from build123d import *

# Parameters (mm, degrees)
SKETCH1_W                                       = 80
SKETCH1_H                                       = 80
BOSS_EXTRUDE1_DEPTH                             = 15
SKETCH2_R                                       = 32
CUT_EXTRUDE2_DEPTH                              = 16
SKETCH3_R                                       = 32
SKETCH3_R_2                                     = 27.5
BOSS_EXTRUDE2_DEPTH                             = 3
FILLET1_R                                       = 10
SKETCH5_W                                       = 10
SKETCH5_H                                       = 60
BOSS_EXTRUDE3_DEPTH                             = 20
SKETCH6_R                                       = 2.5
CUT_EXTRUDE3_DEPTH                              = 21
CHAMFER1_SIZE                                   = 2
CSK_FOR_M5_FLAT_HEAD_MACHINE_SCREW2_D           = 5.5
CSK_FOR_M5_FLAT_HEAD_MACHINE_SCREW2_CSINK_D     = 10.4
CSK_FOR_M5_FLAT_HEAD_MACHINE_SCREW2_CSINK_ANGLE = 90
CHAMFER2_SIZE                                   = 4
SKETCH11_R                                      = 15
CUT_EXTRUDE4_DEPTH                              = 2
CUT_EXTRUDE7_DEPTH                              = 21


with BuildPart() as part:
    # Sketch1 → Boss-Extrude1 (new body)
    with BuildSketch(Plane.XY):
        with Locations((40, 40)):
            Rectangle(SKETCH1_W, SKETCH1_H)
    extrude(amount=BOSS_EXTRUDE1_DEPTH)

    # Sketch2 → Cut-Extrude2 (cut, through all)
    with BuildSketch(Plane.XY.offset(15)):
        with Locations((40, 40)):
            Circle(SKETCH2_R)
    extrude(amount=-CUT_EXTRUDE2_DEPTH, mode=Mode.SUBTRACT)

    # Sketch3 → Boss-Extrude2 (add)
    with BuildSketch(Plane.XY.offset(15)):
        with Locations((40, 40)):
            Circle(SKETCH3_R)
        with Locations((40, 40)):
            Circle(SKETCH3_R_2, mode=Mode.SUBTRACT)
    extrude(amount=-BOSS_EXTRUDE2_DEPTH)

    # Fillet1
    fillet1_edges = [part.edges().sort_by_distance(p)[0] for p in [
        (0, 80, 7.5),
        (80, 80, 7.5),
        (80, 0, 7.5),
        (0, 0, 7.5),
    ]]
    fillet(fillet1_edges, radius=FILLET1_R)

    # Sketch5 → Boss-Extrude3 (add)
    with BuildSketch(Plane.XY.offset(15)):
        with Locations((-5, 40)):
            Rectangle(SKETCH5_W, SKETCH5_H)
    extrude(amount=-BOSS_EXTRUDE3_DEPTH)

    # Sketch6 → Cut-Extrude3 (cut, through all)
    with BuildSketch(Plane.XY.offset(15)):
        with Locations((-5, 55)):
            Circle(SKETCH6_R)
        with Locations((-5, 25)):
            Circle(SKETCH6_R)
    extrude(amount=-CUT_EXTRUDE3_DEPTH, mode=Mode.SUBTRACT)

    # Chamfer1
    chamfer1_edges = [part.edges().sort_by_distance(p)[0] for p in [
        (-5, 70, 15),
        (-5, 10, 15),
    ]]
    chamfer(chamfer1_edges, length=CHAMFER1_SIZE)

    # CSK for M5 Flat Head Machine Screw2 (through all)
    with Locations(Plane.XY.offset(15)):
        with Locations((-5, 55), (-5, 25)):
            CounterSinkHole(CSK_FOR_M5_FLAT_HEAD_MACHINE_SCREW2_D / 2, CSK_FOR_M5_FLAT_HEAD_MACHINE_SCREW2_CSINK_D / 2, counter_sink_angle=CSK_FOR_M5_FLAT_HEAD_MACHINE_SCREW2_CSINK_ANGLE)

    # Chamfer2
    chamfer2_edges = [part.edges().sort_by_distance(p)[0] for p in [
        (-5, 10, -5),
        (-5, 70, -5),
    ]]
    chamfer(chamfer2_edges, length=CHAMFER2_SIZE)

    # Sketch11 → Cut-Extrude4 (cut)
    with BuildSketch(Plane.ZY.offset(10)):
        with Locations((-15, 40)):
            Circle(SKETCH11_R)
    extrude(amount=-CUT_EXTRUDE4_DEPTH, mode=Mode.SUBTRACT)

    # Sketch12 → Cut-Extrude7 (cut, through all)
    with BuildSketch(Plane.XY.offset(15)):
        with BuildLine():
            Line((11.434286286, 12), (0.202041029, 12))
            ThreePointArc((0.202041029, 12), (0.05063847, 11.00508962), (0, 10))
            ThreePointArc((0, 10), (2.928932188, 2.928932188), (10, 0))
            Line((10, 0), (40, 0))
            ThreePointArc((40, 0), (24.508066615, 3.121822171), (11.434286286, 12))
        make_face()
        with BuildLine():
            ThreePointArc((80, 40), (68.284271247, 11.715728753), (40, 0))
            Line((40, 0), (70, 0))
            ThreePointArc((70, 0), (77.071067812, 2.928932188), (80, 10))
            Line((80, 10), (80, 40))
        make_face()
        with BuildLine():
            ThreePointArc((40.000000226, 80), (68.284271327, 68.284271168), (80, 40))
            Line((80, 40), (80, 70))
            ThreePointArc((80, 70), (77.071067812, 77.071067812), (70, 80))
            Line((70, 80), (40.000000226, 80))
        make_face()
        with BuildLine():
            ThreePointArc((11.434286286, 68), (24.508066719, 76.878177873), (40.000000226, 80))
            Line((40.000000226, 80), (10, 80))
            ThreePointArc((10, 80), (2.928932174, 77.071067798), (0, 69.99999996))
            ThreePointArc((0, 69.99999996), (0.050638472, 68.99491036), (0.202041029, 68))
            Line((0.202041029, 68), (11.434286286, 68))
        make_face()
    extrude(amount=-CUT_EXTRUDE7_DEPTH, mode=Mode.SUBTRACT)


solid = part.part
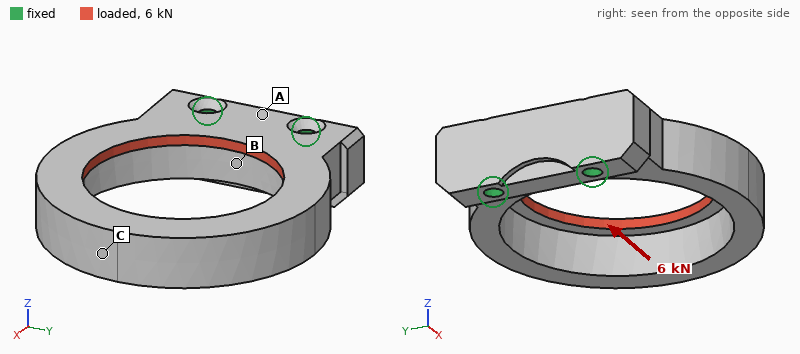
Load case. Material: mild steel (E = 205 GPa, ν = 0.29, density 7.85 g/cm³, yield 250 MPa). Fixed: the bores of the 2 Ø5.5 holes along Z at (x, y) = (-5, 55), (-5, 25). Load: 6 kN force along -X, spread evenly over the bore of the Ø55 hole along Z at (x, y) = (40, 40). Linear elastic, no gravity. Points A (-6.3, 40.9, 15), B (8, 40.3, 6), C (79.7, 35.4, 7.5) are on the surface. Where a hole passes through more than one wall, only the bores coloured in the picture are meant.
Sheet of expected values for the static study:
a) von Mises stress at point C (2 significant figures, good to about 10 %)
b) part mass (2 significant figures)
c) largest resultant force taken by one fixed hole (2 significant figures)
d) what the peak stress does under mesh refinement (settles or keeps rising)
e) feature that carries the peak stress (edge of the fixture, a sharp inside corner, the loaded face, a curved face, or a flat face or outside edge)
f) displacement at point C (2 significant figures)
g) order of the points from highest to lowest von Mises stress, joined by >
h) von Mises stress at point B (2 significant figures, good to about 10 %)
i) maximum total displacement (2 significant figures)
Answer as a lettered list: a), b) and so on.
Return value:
a) 34 MPa
b) 340 g
c) 3.3 kN
d) keeps rising
e) edge of the fixture
f) 79 µm
g) C > B > A
h) 19 MPa
i) 86 µm
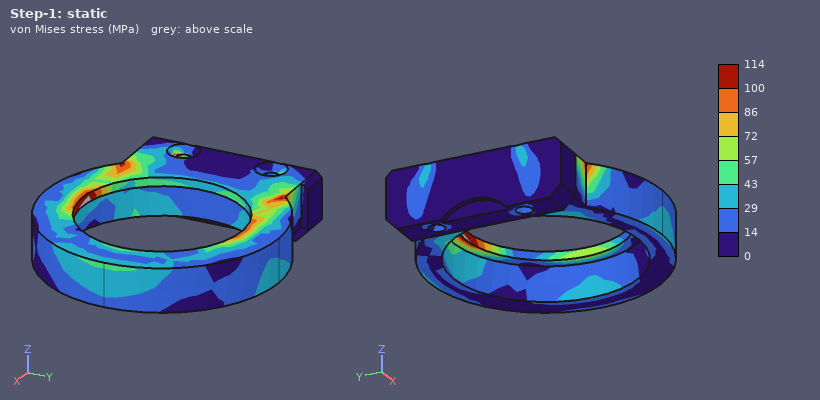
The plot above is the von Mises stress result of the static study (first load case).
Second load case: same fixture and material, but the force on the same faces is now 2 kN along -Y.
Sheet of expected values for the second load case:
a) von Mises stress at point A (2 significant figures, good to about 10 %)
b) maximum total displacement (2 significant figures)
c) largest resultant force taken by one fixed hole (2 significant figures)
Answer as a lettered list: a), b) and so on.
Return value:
a) 8.4 MPa
b) 73 µm
c) 2.5 kN
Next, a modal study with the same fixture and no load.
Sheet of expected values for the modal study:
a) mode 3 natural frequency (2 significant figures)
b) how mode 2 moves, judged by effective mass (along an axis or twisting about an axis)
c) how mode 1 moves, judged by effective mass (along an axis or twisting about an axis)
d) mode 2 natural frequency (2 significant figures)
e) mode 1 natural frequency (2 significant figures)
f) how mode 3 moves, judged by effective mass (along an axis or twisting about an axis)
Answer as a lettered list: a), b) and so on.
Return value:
a) 3300 Hz
b) along Y
c) along Z
d) 1800 Hz
e) 1300 Hz
f) twisting about X
